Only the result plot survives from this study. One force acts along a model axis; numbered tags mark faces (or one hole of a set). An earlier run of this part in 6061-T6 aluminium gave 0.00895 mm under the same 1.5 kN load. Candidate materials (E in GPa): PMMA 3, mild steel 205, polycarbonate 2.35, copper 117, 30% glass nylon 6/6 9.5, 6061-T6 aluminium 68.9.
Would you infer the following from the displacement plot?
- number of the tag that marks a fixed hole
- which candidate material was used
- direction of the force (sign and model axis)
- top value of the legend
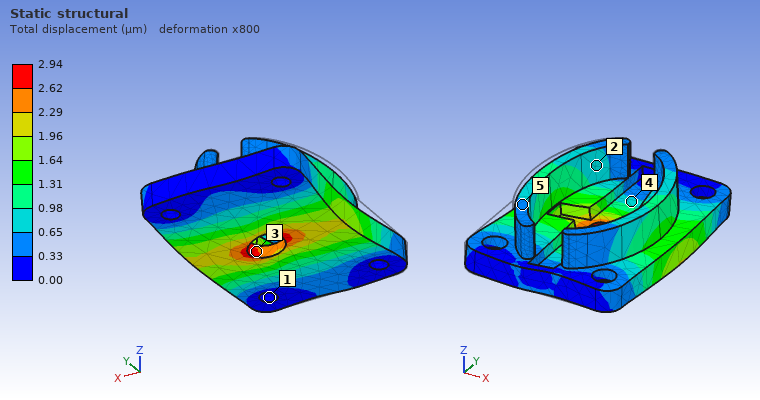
1
mild steel
+X
2.94 µm
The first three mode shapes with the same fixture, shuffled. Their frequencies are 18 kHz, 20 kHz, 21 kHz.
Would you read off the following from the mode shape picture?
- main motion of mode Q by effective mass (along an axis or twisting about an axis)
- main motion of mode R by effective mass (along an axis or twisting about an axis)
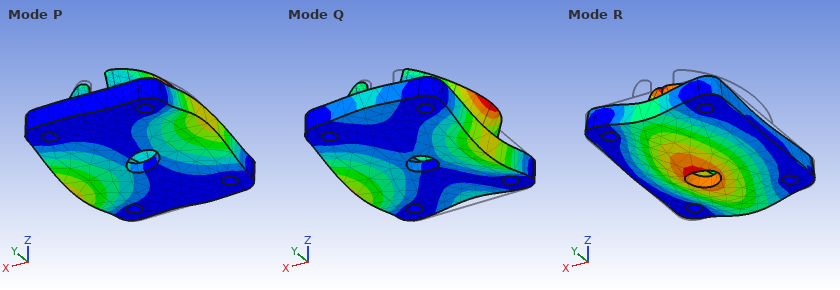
along Z
along Z
